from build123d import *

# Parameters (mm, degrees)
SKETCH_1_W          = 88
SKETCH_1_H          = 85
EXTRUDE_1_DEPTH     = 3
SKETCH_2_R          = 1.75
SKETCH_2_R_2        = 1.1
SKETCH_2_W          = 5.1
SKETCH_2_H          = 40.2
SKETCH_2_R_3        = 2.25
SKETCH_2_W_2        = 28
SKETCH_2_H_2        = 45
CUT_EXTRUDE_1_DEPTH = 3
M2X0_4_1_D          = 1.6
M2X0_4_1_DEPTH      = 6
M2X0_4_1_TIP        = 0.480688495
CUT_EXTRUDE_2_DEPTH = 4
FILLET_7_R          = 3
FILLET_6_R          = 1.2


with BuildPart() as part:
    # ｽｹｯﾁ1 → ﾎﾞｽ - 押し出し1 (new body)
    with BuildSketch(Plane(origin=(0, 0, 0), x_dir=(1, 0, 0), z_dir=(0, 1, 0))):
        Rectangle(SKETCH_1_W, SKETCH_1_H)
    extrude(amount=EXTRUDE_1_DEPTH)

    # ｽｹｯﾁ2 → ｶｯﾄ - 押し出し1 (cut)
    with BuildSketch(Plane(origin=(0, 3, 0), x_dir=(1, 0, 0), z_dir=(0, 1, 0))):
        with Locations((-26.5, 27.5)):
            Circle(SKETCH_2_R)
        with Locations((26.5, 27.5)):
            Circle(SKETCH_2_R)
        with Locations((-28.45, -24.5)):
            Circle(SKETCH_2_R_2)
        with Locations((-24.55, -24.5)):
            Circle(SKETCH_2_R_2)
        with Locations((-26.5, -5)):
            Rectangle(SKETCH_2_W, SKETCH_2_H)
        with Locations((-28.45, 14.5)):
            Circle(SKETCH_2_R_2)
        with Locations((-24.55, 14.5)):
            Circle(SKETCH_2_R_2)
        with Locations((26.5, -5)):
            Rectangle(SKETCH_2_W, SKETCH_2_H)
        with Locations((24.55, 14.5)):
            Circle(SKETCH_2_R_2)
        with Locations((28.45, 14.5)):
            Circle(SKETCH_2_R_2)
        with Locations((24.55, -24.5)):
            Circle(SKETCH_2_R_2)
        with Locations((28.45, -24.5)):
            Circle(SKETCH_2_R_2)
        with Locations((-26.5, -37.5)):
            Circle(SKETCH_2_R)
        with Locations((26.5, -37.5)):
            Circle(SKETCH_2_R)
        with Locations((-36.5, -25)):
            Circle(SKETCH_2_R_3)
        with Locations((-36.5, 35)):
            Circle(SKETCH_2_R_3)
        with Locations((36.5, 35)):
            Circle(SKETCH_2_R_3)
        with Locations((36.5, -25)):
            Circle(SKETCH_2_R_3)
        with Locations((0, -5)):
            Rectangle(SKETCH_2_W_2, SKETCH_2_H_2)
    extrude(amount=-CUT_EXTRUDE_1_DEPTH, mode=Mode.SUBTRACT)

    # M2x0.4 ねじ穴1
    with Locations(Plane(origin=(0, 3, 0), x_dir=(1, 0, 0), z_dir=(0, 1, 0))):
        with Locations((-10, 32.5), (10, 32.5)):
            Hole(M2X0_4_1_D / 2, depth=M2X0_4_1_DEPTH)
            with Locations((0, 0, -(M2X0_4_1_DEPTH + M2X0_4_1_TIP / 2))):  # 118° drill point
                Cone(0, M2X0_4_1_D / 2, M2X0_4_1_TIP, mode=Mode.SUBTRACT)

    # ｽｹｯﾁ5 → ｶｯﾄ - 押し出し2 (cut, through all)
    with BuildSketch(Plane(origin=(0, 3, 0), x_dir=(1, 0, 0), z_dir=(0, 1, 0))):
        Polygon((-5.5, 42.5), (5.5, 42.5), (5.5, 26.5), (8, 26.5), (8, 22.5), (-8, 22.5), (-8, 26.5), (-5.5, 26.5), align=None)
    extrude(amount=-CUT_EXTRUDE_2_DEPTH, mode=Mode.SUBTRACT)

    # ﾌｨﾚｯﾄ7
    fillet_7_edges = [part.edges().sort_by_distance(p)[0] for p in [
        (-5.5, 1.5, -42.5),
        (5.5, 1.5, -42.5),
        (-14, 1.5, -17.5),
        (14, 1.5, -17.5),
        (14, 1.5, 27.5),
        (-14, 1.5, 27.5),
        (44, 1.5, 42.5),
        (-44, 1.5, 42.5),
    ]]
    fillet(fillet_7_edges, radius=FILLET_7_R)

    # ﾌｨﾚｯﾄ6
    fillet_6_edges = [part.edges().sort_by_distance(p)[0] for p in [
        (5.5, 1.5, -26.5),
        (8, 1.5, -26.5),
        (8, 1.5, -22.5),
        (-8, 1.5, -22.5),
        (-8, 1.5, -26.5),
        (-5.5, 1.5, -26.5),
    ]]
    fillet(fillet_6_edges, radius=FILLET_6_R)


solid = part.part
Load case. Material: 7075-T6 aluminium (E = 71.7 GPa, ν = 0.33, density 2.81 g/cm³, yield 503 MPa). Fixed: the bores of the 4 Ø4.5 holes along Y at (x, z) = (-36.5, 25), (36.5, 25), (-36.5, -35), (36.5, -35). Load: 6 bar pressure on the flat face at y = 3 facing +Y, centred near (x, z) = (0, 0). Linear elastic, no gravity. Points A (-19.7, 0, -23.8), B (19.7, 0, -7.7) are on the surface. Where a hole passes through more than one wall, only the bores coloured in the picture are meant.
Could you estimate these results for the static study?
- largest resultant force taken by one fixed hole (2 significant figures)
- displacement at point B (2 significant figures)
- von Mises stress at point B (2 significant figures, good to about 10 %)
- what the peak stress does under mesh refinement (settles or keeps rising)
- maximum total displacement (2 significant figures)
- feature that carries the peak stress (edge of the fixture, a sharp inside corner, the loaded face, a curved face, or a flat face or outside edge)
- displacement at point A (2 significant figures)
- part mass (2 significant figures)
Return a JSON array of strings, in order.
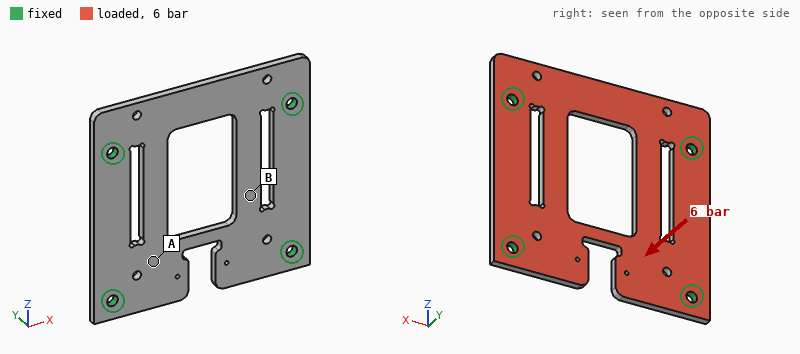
["870 N", "0.37 mm", "62 MPa", "keeps rising", "0.53 mm", "edge of the fixture", "0.26 mm", "46 g"]
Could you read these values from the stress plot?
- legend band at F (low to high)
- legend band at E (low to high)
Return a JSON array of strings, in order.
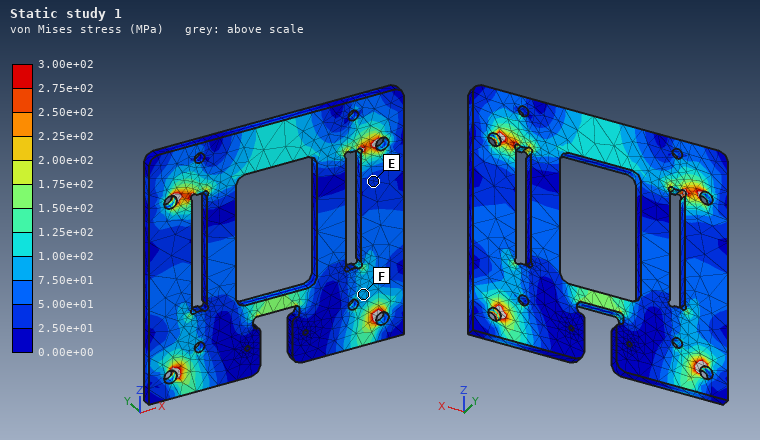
["7.50e+01 to 1.00e+02 MPa", "2.50e+01 to 5.00e+01 MPa"]
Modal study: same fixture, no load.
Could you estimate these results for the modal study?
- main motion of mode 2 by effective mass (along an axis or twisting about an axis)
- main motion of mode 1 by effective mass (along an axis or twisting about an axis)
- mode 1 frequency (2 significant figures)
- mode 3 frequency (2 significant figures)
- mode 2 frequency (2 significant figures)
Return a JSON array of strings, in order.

["twisting about X", "along Y", "2400 Hz", "3700 Hz", "2800 Hz"]
